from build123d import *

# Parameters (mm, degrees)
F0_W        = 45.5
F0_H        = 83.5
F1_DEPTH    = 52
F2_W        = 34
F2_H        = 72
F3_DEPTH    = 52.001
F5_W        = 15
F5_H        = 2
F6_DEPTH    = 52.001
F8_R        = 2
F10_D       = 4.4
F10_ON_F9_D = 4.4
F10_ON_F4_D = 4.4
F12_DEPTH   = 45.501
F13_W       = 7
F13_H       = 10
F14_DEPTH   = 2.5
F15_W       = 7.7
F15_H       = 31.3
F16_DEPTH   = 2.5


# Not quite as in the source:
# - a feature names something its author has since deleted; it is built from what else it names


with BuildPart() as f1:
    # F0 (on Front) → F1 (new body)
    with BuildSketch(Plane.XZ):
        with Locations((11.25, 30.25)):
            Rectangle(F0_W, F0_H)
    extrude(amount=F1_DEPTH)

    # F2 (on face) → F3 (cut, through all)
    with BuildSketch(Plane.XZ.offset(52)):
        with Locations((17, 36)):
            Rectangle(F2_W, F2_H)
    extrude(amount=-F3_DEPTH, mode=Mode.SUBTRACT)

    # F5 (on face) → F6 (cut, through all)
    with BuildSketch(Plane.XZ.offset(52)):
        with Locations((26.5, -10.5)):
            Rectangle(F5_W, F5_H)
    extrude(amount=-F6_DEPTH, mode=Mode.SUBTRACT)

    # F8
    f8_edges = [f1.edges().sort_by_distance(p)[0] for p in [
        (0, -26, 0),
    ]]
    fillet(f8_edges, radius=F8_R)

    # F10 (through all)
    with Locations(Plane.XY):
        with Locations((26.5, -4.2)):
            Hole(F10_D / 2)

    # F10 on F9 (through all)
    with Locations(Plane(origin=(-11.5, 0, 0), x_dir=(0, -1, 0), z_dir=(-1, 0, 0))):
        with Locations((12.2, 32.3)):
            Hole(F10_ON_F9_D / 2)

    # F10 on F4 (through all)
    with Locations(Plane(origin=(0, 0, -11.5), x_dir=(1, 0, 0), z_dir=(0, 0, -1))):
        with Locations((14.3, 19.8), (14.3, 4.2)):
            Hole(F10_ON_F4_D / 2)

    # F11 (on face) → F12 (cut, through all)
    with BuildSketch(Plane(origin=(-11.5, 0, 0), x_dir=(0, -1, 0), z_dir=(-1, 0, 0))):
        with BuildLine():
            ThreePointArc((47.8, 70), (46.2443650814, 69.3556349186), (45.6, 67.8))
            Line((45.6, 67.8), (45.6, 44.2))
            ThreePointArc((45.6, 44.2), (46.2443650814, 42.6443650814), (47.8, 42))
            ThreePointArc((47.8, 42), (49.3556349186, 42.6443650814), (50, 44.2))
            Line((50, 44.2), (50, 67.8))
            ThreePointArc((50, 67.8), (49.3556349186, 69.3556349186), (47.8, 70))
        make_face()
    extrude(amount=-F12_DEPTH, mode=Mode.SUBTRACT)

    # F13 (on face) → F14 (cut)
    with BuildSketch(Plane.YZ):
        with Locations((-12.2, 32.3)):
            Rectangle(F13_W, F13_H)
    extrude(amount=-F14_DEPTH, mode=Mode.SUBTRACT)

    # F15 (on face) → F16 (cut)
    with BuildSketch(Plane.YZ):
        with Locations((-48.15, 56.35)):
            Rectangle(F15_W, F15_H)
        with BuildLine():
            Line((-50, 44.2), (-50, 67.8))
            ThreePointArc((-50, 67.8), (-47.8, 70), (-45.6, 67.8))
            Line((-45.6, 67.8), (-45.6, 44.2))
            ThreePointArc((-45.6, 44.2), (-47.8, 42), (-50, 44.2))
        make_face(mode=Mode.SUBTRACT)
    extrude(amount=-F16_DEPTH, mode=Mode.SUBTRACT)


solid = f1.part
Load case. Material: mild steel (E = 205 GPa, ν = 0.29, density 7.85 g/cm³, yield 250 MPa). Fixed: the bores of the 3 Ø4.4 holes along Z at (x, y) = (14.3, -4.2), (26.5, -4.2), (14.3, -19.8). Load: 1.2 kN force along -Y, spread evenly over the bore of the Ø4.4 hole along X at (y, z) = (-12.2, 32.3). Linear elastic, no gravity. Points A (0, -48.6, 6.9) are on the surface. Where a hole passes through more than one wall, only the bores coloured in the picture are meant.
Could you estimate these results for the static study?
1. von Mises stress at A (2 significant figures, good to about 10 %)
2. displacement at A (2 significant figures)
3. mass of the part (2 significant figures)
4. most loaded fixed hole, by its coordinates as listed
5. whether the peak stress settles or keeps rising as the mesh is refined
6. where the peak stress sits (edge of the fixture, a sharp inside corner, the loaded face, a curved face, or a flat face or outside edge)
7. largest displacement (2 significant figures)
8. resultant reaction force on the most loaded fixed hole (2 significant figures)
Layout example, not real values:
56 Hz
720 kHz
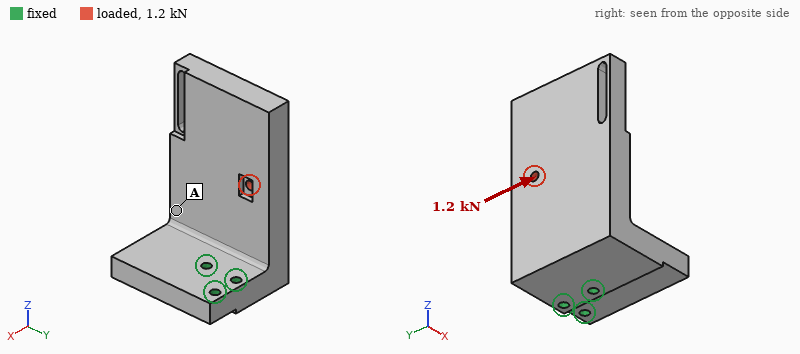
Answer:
9.3 MPa
16 µm
520 g
(14.3, -19.8)
keeps rising
edge of the fixture
41 µm
2.3 kN
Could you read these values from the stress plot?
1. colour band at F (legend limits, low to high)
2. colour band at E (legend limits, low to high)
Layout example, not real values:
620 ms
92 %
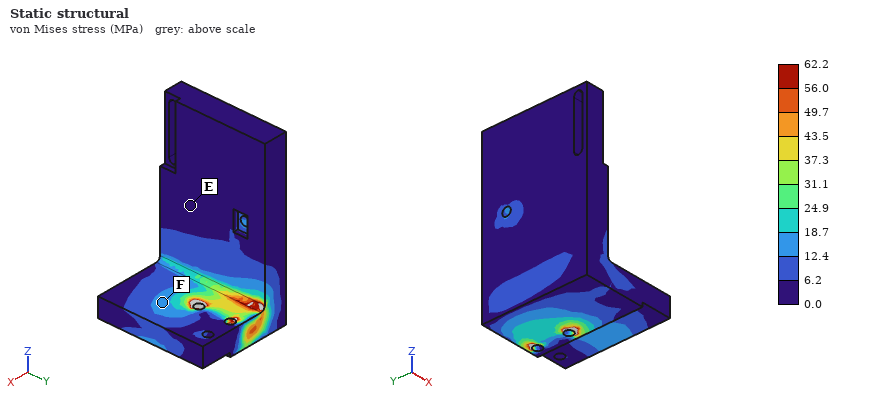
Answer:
12.4 to 18.7 MPa
0.0 to 6.2 MPa
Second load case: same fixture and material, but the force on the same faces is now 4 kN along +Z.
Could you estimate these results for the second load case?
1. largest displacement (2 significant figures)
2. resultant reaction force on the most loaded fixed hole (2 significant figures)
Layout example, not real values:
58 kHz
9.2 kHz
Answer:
88 µm
2.3 kN
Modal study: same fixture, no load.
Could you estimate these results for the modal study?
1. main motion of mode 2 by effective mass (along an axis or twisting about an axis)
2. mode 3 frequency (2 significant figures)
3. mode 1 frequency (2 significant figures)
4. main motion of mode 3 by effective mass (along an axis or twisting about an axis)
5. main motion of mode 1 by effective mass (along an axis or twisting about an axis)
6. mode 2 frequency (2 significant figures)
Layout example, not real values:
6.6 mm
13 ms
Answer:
along Y
4500 Hz
1100 Hz
twisting about Z
along X
1700 Hz
